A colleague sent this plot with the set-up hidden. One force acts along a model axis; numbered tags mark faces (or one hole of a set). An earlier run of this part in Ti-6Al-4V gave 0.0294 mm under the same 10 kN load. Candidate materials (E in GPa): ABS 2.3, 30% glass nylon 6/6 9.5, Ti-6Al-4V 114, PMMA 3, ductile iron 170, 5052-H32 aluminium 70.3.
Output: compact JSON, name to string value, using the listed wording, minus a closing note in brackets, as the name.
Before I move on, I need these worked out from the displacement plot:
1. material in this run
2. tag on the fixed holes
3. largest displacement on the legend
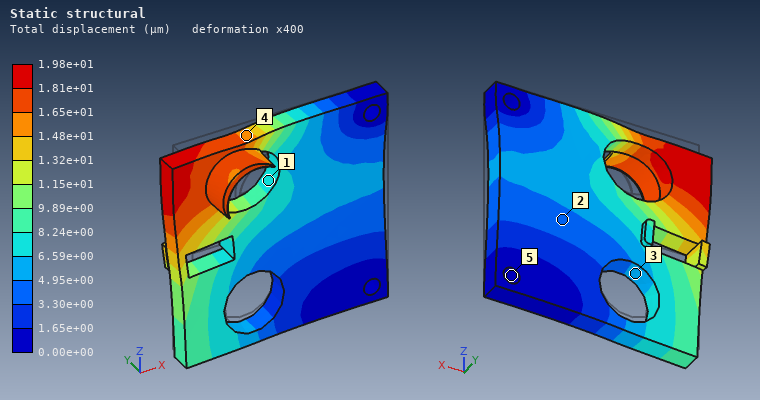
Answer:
{"material in this run": "ductile iron", "tag on the fixed holes": "5", "largest displacement on the legend": "1.98e+01 µm"}
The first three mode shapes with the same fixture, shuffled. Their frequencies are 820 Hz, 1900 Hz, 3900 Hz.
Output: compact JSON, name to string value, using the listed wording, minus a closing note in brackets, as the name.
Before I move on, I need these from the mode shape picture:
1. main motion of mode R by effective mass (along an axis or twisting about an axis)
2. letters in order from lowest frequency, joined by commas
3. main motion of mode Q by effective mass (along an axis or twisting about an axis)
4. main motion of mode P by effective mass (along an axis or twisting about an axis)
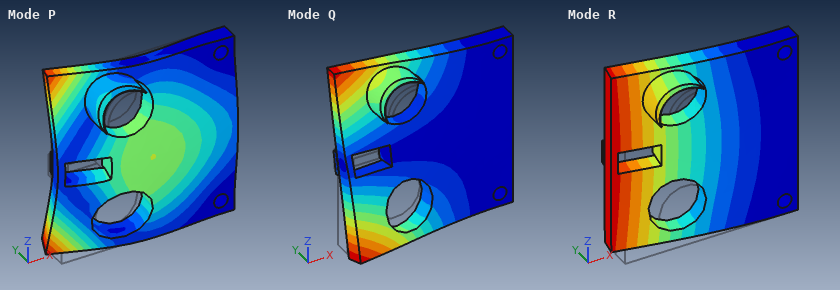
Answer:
{"main motion of mode R by effective mass": "along Y", "letters in order from lowest frequency, joined by commas": "R, Q, P", "main motion of mode Q by effective mass": "twisting about X", "main motion of mode P by effective mass": "along Y"}
